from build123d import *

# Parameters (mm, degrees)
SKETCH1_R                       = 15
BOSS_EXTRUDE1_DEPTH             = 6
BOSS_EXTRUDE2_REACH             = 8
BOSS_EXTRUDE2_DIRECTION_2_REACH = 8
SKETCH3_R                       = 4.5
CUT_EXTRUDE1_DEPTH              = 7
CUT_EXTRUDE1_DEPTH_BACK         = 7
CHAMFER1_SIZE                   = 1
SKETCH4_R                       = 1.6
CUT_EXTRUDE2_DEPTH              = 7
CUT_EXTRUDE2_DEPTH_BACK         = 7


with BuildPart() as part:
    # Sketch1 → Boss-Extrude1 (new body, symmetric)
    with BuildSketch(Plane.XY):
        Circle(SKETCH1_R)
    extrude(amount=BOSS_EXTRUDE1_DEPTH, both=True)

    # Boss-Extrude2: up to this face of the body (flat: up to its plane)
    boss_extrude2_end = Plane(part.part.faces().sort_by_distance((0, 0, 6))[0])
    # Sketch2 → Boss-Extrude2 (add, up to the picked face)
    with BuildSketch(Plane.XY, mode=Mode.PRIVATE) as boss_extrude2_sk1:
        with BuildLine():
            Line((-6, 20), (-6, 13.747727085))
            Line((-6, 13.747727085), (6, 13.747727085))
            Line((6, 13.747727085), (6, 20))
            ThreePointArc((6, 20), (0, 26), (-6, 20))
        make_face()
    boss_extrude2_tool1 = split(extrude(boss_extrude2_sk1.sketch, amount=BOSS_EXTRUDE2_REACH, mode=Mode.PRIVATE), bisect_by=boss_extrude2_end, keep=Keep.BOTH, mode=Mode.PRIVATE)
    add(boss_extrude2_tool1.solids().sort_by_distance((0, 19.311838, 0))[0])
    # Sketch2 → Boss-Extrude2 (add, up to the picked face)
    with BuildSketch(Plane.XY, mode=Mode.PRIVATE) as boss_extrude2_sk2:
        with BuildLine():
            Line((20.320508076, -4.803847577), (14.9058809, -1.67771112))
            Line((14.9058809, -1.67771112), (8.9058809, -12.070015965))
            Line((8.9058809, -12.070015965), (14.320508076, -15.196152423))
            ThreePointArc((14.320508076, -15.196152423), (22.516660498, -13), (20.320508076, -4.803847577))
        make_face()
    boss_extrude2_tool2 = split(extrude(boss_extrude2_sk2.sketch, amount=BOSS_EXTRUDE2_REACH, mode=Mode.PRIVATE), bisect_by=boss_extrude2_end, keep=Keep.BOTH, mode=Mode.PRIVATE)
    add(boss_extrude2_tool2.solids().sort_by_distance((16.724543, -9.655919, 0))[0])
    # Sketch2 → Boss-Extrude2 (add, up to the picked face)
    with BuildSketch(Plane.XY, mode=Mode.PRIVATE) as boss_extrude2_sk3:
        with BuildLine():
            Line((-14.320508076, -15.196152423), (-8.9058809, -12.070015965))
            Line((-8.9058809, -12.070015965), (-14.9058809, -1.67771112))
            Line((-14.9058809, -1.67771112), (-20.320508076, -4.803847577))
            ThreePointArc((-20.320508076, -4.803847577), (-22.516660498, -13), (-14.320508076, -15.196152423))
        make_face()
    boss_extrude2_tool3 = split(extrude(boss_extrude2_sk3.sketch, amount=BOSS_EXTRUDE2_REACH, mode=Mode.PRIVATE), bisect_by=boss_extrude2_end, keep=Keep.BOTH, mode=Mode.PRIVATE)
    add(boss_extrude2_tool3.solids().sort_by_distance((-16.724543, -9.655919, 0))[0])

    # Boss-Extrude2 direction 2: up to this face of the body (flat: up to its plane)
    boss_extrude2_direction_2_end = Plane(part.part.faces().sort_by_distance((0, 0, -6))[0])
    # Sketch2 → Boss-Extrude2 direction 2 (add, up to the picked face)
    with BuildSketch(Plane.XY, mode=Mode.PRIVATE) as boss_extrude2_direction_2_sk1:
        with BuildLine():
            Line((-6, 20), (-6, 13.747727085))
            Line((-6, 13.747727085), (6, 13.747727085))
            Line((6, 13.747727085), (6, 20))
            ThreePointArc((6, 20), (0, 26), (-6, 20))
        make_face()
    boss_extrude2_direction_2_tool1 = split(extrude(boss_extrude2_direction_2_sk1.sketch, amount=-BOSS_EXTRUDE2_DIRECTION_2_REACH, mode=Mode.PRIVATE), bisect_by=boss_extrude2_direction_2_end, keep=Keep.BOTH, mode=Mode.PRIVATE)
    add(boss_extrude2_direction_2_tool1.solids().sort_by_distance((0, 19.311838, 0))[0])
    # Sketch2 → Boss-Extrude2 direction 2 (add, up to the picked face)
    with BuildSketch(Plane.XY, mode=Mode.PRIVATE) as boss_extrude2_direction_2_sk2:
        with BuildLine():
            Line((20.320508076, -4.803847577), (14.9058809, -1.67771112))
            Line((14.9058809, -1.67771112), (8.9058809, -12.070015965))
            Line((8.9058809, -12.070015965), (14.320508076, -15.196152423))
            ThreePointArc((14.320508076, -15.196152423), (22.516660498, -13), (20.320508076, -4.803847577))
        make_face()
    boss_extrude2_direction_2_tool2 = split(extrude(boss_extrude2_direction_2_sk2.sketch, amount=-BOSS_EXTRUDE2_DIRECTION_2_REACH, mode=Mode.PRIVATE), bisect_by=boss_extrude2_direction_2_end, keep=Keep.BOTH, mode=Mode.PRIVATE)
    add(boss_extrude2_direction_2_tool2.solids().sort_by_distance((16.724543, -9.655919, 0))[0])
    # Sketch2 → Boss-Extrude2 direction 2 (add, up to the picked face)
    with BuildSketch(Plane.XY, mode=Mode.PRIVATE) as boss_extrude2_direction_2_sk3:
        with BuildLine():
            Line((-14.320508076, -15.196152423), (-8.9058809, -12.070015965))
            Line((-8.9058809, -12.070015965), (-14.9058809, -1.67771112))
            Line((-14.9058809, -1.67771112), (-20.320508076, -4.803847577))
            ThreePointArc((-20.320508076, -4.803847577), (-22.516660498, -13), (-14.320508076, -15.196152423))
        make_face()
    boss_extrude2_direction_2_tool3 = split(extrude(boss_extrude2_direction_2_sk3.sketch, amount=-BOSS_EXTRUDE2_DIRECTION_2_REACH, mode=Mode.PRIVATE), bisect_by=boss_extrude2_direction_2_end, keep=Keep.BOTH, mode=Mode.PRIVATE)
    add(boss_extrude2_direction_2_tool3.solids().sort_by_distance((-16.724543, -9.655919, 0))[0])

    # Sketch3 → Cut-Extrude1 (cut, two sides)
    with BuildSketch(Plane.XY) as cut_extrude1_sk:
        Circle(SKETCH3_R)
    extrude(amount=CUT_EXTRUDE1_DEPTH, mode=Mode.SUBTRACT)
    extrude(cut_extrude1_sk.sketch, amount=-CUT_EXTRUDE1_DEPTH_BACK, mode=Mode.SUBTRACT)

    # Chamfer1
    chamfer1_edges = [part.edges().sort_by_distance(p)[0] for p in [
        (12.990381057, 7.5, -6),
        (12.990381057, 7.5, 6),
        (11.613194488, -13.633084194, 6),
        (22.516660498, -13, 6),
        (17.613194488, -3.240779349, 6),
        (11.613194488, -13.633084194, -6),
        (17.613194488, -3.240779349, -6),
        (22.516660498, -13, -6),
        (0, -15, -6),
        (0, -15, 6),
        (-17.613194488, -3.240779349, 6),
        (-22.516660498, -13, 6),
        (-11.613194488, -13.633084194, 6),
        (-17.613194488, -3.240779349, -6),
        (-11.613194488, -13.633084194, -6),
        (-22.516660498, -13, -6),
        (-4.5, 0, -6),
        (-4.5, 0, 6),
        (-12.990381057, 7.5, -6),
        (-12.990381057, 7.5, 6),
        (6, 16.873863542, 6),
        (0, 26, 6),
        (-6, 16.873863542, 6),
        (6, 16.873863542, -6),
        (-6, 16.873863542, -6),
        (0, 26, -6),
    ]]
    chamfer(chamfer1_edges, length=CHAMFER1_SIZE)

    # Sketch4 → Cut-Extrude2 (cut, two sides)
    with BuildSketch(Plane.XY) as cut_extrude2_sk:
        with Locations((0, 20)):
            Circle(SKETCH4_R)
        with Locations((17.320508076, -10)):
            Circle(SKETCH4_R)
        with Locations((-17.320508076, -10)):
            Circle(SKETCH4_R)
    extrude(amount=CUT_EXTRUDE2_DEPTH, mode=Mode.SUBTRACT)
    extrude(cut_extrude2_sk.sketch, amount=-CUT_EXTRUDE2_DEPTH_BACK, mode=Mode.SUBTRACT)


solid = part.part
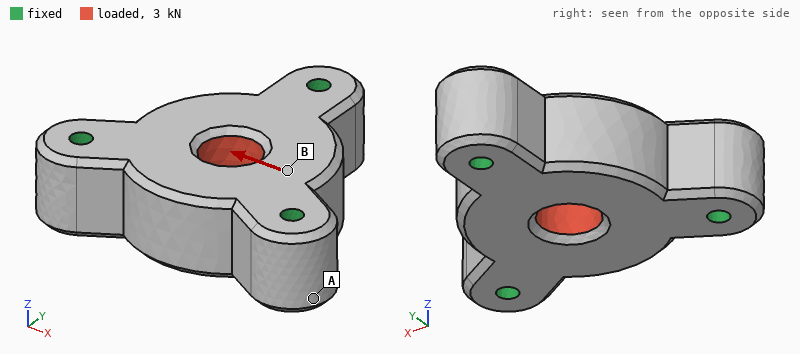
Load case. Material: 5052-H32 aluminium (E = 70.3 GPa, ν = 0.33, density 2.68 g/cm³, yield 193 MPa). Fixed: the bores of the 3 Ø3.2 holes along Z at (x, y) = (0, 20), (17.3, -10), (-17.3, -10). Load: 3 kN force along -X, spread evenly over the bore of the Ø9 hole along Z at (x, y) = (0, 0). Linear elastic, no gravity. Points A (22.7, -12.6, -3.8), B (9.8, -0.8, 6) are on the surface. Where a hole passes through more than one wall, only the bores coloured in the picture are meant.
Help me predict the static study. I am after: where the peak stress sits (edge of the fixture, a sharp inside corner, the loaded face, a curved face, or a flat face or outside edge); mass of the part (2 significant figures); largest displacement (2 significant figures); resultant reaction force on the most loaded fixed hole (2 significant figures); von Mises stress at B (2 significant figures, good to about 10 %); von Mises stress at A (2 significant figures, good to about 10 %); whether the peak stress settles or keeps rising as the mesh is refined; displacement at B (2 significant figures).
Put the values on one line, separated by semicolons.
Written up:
edge of the fixture; 31 g; 4.7 µm; 1.3 kN; 11 MPa; 3.3 MPa; keeps rising; 2.9 µm
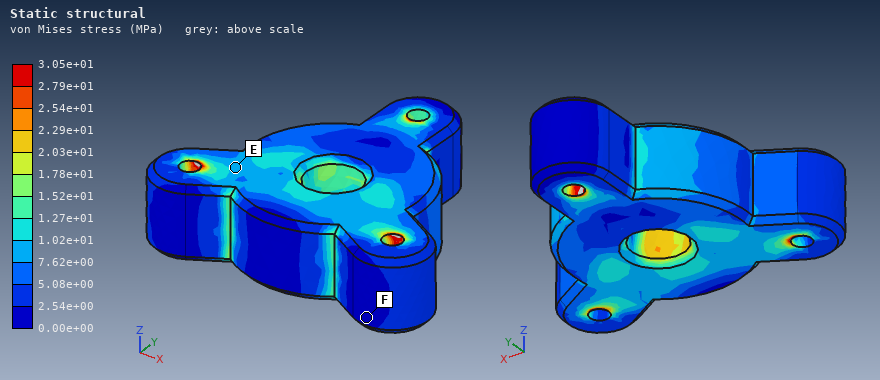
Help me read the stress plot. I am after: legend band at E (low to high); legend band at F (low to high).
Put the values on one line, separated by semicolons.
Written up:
7.62e+00 to 1.02e+01 MPa; 0.00e+00 to 2.54e+00 MPa
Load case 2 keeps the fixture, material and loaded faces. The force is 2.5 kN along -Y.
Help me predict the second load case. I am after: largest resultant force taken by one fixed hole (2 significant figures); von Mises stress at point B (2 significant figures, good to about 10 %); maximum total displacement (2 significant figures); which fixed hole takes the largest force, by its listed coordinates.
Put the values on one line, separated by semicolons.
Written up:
1.2 kN; 3.4 MPa; 4.0 µm; (0, 20)
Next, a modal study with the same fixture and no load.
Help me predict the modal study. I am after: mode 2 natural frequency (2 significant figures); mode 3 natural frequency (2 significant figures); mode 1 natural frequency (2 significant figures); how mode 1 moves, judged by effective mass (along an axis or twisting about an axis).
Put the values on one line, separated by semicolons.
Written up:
35 kHz; 35 kHz; 28 kHz; along Z
